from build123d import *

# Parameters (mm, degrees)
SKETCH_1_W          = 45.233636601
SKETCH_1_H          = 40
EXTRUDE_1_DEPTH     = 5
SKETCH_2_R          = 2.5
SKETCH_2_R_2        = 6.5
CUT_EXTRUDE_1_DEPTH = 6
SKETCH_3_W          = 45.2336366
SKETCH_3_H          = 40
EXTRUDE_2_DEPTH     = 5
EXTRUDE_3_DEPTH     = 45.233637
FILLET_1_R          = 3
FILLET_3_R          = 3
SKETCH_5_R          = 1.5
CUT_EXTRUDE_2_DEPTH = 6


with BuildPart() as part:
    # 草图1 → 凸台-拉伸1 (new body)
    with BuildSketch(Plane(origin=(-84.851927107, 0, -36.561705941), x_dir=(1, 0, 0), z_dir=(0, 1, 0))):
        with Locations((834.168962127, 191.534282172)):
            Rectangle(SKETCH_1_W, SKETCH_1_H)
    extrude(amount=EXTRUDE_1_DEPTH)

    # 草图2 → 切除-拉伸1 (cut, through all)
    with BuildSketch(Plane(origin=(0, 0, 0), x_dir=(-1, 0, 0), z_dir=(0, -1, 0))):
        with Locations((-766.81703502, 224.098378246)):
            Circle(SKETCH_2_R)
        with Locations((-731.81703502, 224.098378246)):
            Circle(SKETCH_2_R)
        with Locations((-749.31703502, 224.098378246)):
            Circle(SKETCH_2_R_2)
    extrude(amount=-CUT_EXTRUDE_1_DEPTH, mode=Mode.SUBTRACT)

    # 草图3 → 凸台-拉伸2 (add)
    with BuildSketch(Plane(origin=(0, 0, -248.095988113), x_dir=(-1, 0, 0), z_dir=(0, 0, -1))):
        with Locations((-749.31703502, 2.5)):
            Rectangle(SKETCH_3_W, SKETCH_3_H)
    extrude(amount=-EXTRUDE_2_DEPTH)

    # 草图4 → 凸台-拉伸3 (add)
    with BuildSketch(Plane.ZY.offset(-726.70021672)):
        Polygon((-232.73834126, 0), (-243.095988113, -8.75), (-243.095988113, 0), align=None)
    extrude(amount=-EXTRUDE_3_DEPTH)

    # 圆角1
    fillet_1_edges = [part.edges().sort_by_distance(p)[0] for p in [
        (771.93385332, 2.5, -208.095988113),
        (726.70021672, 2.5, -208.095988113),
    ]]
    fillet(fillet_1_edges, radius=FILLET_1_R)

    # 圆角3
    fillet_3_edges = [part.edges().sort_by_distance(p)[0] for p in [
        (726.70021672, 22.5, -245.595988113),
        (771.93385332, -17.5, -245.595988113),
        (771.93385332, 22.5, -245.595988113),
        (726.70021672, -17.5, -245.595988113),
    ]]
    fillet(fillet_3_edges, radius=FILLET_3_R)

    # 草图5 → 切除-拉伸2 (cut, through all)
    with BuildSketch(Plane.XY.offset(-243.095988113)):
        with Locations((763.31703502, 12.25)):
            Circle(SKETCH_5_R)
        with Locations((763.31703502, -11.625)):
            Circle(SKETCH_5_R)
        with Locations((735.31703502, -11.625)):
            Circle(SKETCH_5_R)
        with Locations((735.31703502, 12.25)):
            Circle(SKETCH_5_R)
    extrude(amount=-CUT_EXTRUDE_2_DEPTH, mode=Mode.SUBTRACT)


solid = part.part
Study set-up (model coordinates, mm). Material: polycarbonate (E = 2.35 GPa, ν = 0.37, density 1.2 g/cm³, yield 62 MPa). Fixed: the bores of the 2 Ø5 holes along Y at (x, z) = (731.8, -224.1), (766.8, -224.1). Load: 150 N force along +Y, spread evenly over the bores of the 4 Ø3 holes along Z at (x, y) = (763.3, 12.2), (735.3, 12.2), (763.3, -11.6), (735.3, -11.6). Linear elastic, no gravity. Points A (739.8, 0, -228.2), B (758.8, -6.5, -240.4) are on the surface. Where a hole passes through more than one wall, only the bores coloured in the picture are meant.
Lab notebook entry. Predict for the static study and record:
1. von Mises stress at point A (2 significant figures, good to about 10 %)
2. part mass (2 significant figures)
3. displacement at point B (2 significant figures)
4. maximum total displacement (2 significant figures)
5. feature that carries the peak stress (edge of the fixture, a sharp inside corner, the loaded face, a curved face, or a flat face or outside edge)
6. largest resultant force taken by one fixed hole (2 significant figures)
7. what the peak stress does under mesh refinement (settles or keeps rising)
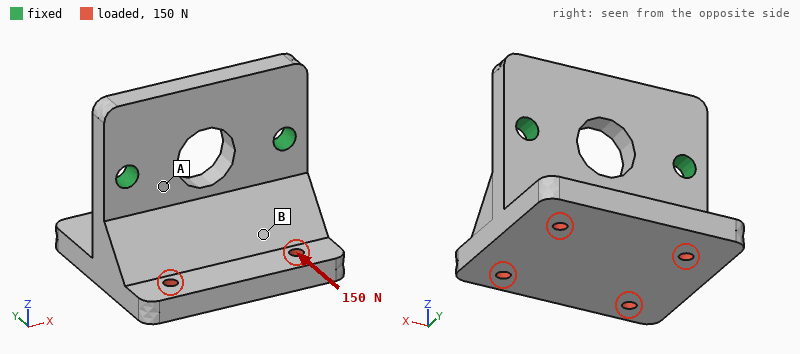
12 MPa
22 g
0.41 mm
0.79 mm
edge of the fixture
75 N
keeps rising
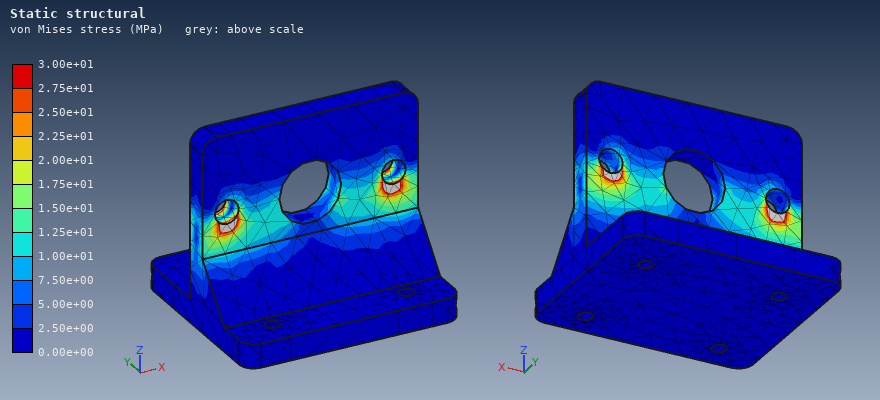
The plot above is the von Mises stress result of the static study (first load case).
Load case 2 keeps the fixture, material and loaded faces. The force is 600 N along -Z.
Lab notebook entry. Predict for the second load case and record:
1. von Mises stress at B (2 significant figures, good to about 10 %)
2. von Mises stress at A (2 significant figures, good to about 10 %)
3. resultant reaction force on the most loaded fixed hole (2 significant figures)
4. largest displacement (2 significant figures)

4.3 MPa
8.7 MPa
300 N
0.48 mm
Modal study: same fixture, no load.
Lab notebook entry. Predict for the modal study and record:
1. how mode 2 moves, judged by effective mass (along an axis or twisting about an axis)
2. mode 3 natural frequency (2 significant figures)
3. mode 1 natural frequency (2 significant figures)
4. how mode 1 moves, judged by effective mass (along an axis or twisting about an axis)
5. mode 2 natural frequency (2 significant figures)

twisting about Z
2600 Hz
660 Hz
along Y
1800 Hz
